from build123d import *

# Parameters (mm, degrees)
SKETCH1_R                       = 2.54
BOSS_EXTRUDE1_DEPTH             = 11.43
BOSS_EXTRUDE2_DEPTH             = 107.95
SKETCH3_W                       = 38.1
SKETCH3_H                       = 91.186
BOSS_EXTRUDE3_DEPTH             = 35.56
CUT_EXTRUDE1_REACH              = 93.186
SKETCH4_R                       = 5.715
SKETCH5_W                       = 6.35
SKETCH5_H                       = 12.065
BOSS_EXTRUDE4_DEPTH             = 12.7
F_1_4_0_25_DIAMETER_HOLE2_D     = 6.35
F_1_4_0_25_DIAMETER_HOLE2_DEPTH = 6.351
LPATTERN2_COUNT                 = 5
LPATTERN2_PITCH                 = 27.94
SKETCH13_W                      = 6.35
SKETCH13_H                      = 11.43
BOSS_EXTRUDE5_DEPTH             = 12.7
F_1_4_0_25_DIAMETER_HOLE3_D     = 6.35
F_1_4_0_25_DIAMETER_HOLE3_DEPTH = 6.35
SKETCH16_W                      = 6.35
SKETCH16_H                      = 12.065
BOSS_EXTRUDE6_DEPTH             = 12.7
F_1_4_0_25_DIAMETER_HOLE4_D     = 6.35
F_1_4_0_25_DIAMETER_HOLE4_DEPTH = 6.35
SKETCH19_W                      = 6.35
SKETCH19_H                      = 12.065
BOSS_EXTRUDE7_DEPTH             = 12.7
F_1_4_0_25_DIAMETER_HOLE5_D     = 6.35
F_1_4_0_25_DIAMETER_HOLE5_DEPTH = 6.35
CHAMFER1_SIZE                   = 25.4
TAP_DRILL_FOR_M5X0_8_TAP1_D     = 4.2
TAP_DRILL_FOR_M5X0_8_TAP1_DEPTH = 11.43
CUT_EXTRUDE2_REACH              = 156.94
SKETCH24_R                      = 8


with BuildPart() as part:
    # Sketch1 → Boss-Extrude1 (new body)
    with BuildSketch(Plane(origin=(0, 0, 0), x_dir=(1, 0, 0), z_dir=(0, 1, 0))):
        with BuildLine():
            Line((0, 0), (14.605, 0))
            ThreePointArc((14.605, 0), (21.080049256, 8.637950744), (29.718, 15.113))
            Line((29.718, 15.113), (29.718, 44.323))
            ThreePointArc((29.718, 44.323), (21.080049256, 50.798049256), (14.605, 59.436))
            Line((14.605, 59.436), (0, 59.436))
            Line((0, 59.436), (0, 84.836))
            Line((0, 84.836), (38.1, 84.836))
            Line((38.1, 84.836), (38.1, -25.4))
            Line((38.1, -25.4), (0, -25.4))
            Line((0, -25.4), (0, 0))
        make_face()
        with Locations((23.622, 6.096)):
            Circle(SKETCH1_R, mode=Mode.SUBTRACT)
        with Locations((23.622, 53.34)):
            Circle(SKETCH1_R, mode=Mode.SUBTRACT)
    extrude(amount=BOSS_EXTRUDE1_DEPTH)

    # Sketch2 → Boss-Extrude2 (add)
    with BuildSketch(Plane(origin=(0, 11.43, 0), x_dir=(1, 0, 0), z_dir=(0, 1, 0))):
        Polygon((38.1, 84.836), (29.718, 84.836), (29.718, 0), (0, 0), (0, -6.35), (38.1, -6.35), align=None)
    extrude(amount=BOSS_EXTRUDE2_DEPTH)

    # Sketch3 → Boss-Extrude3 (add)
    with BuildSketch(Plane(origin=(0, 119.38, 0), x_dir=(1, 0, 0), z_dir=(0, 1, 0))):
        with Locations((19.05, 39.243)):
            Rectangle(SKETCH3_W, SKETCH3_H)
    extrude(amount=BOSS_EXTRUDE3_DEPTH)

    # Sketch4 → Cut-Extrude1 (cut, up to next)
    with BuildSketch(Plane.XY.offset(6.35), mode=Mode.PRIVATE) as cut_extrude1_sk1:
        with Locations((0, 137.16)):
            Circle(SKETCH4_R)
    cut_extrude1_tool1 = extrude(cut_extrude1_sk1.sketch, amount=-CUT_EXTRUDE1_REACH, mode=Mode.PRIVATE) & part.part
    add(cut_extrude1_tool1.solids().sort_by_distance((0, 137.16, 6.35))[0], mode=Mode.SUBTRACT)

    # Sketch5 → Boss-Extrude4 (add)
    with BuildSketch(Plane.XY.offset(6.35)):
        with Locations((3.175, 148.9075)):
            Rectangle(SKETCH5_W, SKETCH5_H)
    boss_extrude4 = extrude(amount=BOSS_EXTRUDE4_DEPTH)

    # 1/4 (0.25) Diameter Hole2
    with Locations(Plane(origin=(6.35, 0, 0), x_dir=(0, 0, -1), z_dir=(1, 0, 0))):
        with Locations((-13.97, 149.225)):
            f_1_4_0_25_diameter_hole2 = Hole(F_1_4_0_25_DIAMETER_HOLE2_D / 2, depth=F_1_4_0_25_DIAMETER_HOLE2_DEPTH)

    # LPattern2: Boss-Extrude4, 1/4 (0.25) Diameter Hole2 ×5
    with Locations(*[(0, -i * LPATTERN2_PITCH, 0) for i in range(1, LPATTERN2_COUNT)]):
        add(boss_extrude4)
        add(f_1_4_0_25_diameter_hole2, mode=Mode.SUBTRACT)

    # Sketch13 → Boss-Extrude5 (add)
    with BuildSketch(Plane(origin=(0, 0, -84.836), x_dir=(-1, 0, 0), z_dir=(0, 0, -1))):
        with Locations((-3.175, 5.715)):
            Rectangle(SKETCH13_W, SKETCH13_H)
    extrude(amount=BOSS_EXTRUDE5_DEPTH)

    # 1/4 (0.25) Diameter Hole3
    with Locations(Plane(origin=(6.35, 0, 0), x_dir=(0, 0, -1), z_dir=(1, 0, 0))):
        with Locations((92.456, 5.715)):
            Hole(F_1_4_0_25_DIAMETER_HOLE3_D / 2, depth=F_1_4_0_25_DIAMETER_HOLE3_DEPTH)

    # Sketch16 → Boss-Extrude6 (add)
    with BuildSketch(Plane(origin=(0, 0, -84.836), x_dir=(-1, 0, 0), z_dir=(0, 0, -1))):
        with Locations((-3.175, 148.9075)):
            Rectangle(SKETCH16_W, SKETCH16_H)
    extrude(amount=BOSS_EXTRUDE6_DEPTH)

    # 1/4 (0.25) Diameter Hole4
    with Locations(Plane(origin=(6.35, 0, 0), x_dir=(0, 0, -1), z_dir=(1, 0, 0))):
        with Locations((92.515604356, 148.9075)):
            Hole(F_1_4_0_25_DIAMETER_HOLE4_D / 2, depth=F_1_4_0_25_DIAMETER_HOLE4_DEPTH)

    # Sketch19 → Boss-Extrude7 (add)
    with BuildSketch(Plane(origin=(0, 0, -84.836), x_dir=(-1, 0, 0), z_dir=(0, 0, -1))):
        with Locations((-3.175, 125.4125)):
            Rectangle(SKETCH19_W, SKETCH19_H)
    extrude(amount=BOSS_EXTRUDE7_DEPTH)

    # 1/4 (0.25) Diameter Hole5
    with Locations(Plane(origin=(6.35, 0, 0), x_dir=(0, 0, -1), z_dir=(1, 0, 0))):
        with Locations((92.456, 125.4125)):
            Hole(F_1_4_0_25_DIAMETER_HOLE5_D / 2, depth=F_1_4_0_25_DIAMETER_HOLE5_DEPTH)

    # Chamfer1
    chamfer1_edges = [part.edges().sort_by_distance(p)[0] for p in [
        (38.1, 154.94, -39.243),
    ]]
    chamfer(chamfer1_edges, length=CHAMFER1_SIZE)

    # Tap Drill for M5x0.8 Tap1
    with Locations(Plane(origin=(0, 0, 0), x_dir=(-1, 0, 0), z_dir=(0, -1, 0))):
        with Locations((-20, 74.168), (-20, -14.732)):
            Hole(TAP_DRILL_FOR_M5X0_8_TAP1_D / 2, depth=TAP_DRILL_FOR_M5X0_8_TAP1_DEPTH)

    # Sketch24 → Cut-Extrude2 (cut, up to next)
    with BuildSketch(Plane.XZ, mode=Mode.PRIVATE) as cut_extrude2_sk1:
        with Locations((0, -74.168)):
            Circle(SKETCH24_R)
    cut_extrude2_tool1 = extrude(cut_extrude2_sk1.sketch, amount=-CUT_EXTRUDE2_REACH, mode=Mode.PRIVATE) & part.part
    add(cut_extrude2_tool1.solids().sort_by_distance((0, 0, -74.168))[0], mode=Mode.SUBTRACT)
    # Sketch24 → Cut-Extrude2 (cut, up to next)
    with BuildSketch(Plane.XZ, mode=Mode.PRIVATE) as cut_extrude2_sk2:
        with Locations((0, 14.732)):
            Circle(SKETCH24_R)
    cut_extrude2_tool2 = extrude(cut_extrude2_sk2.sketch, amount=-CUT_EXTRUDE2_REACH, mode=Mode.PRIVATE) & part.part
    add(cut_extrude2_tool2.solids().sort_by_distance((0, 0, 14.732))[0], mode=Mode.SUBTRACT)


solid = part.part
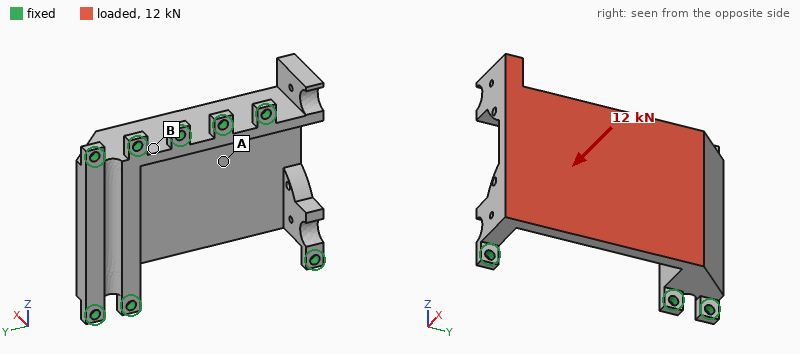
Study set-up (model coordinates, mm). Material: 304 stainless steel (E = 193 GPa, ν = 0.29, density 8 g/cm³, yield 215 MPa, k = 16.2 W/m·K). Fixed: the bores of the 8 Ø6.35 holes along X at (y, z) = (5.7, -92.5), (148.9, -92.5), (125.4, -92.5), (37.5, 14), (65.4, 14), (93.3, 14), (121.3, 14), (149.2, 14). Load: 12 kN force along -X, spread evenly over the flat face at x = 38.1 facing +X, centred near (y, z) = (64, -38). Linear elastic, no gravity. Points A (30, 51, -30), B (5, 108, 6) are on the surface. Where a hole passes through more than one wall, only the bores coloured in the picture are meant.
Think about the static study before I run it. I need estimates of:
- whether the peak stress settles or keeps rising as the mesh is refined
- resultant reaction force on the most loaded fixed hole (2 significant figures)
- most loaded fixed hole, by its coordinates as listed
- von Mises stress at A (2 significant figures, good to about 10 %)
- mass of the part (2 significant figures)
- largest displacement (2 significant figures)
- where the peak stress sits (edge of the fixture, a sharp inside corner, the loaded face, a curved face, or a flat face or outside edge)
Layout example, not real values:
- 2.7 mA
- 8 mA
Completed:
- keeps rising
- 3.7 kN
- (5.7, -92.5)
- 21 MPa
- 1.8 kg
- 80 µm
- edge of the fixture
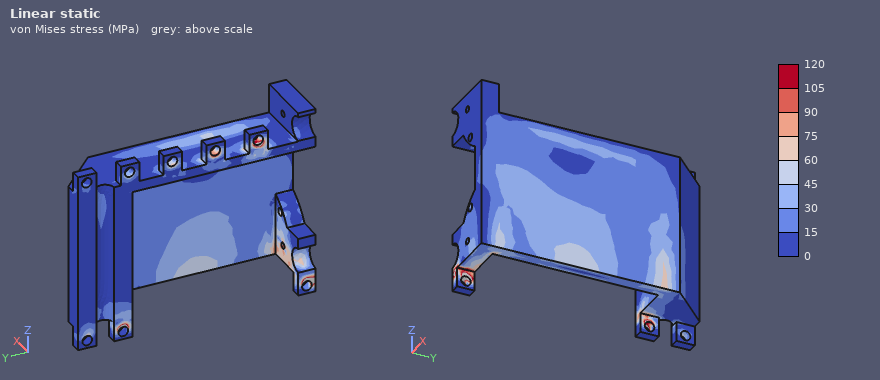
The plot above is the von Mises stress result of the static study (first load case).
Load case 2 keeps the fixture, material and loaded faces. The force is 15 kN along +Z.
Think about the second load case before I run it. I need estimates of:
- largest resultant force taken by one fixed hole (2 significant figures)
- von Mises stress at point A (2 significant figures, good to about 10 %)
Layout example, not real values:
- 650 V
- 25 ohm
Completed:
- 4.0 kN
- 12 MPa
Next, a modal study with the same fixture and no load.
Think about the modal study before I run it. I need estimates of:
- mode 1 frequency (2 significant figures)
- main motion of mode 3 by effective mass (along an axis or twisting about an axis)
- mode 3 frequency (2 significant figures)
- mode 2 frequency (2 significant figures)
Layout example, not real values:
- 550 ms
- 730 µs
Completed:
- 2600 Hz
- along Y
- 3400 Hz
- 3000 Hz
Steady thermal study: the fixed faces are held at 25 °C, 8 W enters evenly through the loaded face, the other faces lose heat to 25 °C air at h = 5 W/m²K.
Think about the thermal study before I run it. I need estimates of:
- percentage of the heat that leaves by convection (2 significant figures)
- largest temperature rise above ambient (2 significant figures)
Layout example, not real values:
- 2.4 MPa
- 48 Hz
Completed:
- 26 %
- 19 K
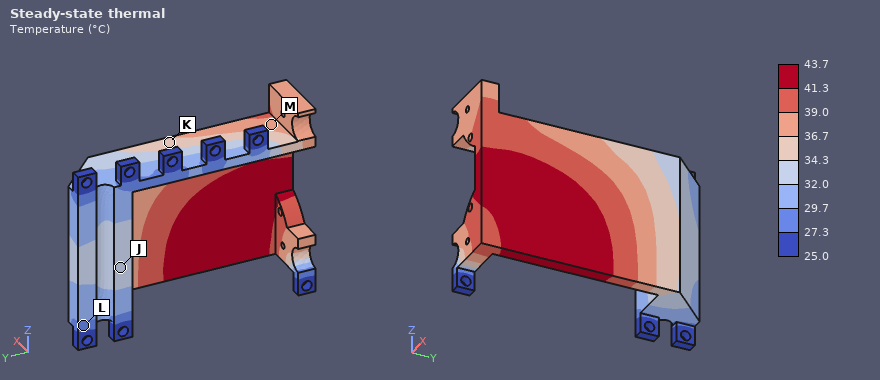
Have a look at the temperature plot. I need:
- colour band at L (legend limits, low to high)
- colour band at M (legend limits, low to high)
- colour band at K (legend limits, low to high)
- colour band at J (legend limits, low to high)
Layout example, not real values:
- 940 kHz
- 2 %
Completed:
- 27.3 to 29.7 °C
- 36.7 to 39.0 °C
- 34.3 to 36.7 °C
- 32.0 to 34.3 °C
